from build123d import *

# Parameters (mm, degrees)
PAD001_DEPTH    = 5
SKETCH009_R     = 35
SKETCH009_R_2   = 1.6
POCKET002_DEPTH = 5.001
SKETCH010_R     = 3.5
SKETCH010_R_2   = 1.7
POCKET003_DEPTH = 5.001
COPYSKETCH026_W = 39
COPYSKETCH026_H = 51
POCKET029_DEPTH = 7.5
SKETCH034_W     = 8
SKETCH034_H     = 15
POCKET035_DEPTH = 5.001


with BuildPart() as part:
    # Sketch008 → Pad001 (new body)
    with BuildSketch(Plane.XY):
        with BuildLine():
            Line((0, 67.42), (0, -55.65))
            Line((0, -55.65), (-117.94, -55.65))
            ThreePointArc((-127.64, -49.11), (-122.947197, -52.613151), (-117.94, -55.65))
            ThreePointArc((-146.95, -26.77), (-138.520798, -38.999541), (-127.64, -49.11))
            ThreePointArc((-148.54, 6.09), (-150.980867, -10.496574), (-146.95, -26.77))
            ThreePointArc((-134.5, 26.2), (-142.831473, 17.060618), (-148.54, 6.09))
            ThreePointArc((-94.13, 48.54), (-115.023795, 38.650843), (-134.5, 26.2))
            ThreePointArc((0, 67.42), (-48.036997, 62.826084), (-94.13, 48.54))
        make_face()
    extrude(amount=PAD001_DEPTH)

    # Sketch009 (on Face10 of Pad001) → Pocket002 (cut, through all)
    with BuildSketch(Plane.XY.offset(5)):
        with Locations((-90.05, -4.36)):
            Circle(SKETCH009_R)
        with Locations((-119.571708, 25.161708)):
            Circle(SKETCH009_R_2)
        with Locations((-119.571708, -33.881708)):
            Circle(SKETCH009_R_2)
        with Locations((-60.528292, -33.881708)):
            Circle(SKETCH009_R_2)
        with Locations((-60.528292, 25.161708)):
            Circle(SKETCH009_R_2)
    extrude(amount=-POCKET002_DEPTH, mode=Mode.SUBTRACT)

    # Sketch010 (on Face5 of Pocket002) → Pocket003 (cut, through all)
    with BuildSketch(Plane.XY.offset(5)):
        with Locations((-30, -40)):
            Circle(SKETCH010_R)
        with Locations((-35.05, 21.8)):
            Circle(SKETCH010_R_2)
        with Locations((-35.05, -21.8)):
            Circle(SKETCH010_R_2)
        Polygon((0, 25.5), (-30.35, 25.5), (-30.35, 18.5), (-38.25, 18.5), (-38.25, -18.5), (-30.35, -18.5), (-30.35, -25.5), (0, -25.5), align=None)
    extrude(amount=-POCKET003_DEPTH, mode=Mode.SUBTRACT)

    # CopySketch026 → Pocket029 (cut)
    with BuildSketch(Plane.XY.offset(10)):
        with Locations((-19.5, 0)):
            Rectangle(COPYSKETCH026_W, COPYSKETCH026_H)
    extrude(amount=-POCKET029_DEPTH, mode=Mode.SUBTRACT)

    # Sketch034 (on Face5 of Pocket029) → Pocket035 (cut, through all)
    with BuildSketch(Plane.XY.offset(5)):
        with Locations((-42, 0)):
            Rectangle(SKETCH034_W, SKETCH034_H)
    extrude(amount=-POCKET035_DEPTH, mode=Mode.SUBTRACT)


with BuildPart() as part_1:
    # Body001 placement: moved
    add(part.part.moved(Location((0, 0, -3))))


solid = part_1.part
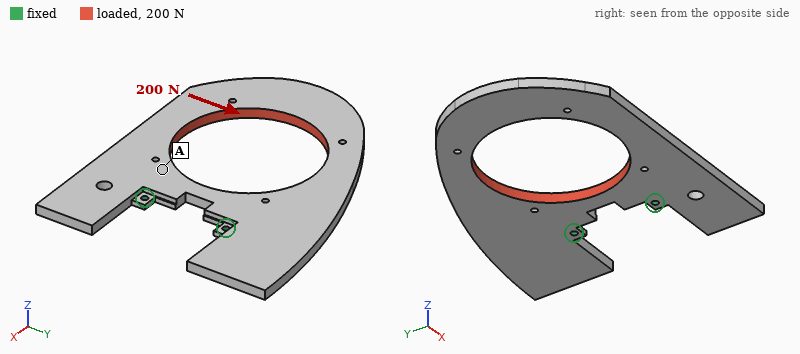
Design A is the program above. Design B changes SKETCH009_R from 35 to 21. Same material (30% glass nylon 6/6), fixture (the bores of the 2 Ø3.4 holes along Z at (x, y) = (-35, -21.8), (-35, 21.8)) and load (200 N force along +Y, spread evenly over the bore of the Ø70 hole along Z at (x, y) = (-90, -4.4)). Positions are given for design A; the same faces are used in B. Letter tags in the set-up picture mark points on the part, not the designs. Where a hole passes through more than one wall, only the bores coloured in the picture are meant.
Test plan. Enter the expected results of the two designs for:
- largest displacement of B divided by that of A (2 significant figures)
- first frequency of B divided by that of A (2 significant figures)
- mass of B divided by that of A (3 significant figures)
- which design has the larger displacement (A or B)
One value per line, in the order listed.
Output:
0.39
0.95
1.26
A
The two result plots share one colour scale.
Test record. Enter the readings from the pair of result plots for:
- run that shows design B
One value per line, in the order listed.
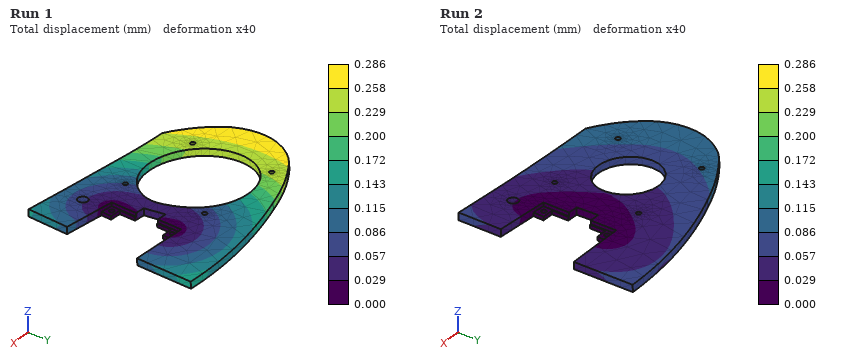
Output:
Run 2
